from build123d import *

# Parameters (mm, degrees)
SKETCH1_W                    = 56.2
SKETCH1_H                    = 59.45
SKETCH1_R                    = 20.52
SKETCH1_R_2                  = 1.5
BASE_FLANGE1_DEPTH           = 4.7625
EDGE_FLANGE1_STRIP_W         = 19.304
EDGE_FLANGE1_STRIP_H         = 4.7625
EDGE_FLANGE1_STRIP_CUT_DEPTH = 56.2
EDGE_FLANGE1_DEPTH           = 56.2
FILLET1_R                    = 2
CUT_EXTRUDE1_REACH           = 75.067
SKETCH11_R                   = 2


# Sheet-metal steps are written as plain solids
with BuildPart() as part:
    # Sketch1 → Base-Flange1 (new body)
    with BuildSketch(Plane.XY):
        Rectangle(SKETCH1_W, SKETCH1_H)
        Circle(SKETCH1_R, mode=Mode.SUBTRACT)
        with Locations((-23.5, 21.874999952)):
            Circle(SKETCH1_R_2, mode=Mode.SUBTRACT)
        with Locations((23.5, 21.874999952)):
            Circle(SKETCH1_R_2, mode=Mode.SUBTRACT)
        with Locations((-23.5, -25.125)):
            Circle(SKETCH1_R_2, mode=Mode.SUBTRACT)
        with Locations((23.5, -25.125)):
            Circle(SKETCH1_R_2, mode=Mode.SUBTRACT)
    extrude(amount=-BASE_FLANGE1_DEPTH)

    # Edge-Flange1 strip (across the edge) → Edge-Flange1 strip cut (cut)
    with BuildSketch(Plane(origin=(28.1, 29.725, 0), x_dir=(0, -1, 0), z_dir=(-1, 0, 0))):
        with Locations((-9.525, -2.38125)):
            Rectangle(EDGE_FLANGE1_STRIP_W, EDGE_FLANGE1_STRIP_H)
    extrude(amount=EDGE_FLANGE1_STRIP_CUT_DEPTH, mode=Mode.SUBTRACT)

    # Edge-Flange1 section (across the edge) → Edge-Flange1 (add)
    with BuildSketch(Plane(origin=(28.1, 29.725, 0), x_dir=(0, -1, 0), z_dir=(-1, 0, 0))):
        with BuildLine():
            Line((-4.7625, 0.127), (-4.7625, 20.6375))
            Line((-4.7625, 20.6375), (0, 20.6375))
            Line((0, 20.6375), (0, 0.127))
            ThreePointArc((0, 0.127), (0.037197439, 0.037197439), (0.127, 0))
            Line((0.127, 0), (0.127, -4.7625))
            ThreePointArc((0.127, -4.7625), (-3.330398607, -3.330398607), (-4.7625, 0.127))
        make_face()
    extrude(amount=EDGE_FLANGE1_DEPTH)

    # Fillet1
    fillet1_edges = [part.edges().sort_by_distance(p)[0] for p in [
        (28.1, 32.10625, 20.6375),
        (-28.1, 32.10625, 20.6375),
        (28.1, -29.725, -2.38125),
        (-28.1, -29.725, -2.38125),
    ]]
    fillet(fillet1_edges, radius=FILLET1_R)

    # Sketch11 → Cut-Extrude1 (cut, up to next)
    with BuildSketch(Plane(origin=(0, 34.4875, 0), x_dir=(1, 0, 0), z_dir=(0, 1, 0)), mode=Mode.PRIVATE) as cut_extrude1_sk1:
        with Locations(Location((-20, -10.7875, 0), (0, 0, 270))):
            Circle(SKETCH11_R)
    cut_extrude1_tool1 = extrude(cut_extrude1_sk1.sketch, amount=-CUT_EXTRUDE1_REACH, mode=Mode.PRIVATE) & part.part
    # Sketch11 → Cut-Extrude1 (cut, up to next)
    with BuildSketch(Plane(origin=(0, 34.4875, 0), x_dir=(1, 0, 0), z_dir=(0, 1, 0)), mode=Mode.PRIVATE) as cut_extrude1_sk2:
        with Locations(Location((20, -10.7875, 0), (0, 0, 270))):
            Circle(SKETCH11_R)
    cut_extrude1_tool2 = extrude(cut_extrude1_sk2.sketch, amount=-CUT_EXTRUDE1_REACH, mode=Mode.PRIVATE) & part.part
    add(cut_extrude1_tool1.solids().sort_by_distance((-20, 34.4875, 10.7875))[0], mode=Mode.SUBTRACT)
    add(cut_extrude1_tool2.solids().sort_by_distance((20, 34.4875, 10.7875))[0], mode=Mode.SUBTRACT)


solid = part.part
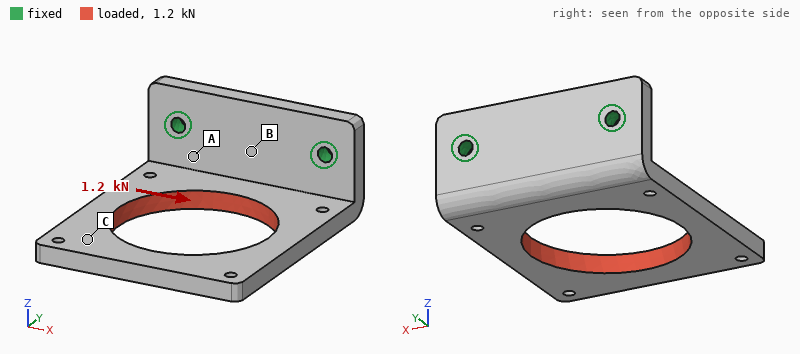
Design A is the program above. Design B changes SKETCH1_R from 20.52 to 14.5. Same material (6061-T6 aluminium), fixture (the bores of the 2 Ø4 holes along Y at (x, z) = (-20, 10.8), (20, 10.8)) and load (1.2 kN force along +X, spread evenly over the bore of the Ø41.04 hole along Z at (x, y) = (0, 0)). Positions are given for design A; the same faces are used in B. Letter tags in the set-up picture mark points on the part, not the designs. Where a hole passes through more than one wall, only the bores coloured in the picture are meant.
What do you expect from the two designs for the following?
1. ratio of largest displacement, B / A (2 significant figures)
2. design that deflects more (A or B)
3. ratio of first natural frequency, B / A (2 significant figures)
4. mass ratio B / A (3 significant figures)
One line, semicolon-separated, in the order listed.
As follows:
0.74; A; 1.0; 1.20
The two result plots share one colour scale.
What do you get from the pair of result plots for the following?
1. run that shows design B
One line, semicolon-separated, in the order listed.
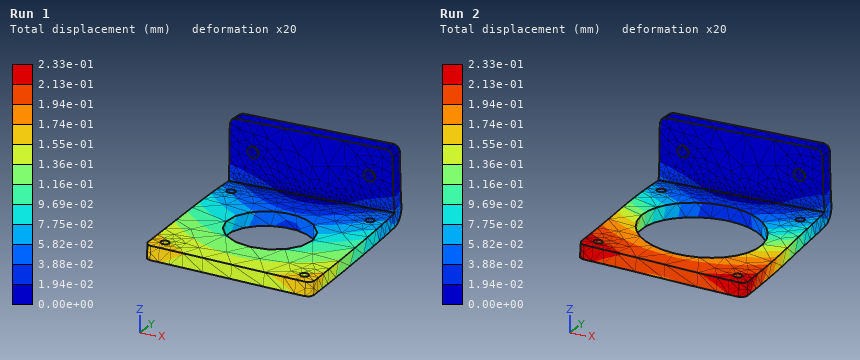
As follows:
Run 1
